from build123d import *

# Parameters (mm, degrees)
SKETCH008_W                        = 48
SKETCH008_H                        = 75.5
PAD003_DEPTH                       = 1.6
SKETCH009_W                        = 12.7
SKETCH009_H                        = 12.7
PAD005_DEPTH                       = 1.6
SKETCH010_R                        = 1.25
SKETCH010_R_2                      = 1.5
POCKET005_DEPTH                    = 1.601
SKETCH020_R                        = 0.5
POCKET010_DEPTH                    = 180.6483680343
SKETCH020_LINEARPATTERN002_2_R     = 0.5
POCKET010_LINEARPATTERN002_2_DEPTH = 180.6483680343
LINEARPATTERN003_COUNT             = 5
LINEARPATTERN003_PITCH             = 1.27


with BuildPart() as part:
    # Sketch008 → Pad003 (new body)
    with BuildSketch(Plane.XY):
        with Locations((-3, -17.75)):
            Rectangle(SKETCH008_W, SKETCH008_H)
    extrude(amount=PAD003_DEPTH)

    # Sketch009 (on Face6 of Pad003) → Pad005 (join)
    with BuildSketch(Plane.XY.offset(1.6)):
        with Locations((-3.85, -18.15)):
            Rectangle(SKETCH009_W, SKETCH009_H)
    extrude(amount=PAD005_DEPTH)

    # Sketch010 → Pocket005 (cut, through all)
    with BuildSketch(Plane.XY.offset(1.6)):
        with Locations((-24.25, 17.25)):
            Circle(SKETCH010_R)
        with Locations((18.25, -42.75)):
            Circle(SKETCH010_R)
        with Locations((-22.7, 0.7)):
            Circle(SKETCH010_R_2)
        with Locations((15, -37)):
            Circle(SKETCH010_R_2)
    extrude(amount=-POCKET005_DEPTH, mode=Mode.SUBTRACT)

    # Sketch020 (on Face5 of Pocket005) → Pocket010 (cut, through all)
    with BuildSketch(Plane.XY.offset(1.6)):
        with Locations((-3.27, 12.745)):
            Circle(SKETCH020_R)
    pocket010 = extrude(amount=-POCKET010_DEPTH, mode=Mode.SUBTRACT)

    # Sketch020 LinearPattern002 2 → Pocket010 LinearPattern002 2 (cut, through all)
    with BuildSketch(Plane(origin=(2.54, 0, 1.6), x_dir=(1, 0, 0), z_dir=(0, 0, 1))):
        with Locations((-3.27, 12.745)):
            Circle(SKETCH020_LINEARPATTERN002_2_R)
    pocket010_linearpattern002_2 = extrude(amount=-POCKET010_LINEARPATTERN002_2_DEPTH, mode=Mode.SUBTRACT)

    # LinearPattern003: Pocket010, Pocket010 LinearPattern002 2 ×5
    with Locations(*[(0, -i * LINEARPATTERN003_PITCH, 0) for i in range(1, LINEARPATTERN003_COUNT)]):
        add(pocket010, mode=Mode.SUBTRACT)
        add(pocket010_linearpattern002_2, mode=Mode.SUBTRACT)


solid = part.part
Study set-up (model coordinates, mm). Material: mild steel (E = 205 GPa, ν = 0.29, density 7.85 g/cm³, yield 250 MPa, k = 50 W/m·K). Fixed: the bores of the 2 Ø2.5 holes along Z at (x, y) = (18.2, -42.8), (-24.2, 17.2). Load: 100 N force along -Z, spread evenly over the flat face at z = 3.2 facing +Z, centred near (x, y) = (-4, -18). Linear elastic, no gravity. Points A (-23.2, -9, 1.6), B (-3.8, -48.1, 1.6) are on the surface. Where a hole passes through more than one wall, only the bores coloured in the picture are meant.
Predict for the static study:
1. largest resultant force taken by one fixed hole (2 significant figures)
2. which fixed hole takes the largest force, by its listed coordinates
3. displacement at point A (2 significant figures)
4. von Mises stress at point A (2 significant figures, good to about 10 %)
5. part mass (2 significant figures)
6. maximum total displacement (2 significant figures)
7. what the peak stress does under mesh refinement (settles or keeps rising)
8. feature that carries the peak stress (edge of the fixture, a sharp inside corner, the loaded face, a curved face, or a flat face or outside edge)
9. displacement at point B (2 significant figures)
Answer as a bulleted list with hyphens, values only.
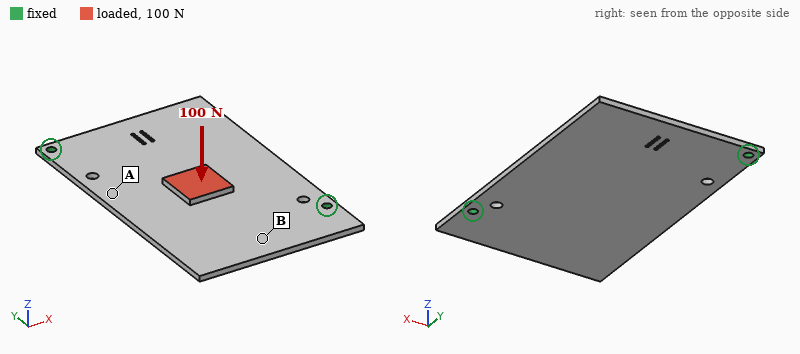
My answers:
- 63 N
- (18.2, -42.8)
- 0.087 mm
- 33 MPa
- 47 g
- 0.13 mm
- keeps rising
- edge of the fixture
- 0.049 mm
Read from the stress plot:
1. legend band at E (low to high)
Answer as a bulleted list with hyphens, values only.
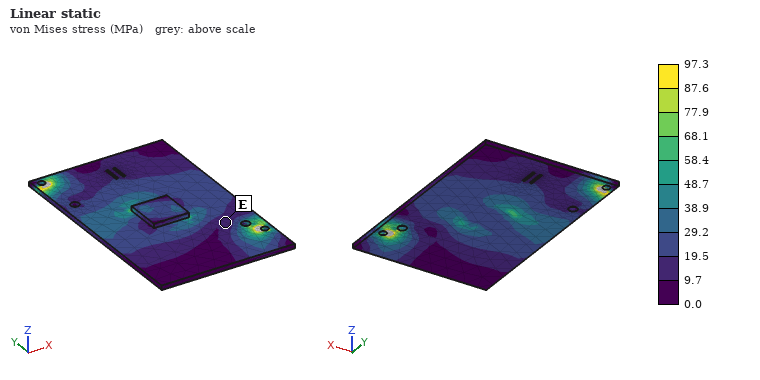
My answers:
- 9.7 to 19.5 MPa
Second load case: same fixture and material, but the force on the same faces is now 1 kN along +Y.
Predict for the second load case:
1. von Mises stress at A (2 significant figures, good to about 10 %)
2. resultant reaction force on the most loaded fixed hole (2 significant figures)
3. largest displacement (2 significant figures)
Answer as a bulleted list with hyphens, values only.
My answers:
- 46 MPa
- 510 N
- 0.25 mm
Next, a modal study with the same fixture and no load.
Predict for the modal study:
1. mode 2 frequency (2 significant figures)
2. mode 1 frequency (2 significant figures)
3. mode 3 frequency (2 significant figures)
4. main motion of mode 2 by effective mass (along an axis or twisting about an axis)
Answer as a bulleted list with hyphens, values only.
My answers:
- 950 Hz
- 670 Hz
- 1900 Hz
- along Z
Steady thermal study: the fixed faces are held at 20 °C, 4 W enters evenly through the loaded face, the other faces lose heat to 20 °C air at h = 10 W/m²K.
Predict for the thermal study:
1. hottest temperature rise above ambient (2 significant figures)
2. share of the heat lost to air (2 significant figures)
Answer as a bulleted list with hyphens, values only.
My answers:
- 29 K
- 32 %
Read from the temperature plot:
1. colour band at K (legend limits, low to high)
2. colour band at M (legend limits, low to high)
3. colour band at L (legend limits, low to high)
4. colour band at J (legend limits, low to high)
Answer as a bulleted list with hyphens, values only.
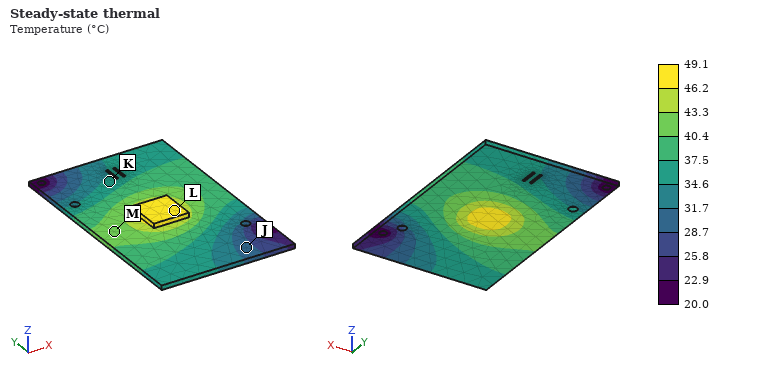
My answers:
- 34.6 to 37.5 °C
- 40.4 to 43.3 °C
- 46.2 to 49.1 °C
- 28.7 to 31.7 °C
